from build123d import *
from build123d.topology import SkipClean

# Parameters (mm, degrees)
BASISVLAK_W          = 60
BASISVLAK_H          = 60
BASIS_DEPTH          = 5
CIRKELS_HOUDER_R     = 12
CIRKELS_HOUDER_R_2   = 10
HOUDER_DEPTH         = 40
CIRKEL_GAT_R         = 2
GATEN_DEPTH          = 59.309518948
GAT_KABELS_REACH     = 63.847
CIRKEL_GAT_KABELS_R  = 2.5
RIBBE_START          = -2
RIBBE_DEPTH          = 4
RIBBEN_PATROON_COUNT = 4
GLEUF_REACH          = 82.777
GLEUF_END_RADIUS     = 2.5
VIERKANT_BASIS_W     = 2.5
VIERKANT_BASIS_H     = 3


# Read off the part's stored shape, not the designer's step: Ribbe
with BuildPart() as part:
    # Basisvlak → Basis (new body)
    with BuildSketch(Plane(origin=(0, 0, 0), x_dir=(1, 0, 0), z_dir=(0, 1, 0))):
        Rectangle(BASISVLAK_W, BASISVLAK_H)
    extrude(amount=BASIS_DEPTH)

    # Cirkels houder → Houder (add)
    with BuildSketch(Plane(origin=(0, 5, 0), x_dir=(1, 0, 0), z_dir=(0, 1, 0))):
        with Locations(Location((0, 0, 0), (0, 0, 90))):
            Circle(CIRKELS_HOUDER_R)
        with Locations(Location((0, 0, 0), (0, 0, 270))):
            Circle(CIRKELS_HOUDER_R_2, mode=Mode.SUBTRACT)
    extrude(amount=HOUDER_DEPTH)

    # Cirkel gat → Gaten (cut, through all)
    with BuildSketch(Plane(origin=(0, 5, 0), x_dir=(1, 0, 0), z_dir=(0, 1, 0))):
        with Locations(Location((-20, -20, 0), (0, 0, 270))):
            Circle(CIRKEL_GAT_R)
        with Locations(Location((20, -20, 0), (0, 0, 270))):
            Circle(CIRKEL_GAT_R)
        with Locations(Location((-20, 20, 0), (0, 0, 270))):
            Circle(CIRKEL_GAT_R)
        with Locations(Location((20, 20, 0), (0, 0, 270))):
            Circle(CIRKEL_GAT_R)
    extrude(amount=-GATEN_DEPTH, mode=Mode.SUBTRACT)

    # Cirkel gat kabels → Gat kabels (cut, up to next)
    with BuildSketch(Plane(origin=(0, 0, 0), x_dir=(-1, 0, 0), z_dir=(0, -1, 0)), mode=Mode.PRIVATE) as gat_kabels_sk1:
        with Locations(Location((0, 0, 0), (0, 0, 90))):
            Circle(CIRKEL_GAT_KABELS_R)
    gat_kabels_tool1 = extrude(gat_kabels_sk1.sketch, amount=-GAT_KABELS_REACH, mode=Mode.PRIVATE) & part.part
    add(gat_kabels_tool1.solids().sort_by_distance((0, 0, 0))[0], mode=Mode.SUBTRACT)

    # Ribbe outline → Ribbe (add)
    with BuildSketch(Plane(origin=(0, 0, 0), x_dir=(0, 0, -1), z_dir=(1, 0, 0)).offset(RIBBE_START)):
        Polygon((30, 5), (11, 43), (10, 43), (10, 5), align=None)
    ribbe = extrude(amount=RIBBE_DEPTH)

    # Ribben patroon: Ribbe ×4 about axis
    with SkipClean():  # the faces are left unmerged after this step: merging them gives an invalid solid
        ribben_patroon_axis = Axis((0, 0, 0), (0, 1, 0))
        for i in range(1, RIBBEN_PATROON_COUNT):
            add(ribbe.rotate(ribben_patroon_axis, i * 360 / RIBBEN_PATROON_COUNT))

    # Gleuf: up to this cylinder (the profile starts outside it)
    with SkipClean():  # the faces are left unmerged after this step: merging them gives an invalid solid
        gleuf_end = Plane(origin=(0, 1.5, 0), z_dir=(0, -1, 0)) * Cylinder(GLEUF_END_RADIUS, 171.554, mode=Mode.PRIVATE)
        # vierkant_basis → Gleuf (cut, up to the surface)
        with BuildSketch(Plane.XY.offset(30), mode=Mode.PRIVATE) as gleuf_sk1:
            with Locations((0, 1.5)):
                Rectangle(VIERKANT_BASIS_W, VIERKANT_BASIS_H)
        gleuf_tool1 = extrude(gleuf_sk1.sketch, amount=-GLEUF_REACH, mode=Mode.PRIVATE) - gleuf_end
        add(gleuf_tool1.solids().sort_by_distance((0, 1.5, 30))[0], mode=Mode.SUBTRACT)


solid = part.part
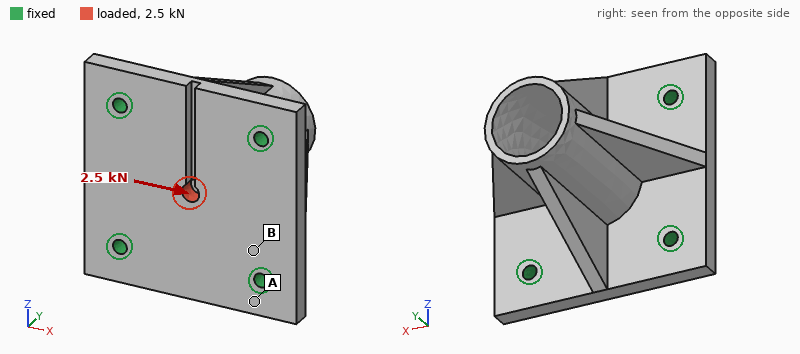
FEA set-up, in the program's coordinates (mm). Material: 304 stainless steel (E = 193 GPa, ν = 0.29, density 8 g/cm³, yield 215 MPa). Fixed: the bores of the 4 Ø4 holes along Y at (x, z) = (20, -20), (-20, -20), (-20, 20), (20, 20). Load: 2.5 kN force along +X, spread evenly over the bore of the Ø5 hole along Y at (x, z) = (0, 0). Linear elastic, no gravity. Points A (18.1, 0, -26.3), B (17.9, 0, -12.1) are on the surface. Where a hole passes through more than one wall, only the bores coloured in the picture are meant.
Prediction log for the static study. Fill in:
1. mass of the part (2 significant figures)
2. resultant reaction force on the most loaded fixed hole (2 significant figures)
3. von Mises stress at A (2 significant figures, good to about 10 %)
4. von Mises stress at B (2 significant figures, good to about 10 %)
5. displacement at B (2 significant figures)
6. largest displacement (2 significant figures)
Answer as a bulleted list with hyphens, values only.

- 230 g
- 730 N
- 2.9 MPa
- 9.4 MPa
- 0.66 µm
- 2.3 µm
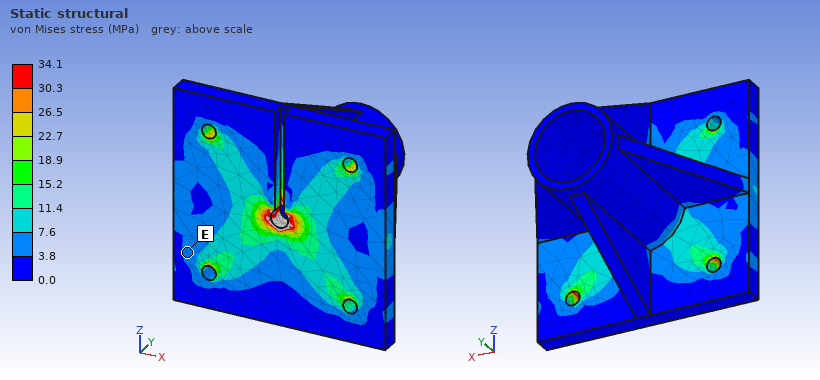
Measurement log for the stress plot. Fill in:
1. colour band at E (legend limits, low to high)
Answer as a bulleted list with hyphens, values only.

- 3.8 to 7.6 MPa
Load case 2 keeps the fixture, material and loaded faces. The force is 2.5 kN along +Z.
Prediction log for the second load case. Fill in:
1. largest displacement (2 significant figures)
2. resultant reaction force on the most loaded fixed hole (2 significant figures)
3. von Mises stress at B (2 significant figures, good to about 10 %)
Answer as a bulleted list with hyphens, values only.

- 2.3 µm
- 690 N
- 8.3 MPa
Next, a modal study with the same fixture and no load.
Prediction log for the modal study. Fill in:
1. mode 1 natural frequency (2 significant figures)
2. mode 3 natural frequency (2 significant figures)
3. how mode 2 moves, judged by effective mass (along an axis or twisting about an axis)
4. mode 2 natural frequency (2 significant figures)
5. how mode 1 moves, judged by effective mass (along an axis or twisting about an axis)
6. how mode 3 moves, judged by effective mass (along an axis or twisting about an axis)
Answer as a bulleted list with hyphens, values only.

- 6100 Hz
- 8000 Hz
- along X
- 6500 Hz
- along Z
- along Y
